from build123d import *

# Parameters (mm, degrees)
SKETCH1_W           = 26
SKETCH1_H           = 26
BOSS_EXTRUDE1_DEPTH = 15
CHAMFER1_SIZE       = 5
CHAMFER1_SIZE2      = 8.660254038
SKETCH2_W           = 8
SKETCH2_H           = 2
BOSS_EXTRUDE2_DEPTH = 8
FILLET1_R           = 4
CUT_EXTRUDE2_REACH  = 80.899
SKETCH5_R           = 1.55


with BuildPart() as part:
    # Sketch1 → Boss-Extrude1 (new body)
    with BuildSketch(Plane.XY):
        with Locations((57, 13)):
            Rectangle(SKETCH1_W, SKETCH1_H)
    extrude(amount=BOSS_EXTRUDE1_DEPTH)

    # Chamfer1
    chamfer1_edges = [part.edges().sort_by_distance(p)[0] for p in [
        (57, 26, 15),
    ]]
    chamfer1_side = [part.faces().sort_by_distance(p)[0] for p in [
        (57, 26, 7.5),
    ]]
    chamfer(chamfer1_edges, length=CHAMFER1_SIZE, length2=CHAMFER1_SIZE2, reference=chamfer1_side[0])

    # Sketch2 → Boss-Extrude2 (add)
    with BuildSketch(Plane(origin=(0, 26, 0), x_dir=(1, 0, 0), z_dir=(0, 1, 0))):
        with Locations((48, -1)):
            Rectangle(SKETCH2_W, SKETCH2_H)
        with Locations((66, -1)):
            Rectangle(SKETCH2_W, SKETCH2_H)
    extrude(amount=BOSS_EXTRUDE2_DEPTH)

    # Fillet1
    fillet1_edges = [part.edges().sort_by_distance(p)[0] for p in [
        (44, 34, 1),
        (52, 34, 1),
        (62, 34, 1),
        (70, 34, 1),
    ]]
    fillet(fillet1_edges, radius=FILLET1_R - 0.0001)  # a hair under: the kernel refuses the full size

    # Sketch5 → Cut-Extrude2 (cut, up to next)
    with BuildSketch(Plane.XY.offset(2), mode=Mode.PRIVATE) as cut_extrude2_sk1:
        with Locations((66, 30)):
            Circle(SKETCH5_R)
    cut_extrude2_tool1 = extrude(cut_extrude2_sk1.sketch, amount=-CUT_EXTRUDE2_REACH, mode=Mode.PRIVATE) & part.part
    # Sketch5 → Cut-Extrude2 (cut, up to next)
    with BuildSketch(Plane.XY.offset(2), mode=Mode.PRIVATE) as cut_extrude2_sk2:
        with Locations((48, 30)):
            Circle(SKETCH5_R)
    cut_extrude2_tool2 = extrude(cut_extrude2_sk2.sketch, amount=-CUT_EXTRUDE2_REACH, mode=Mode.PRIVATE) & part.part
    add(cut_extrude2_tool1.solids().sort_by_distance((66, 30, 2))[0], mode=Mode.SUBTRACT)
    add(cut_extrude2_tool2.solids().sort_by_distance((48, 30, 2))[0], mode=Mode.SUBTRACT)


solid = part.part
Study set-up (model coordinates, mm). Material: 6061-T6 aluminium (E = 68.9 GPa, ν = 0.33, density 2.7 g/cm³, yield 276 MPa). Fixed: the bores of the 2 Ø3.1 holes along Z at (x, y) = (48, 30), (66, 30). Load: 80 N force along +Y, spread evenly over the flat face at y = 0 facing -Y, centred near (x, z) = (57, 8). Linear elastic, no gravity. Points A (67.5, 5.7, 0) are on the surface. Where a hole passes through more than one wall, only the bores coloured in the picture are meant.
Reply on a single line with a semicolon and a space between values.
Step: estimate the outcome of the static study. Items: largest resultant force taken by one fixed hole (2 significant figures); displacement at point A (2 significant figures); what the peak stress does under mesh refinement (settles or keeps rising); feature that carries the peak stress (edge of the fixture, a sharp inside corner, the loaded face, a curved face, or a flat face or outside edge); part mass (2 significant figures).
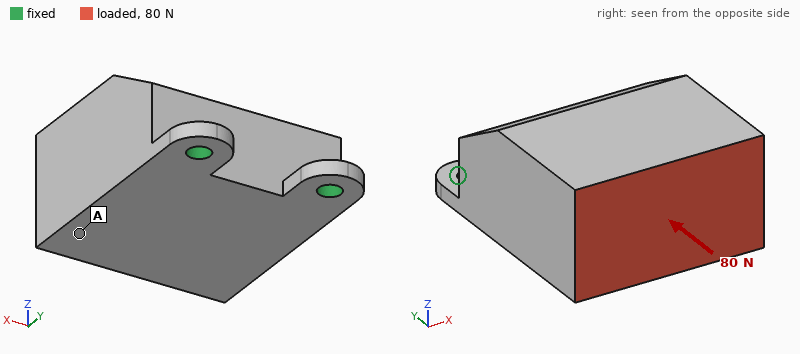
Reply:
40 N; 59 µm; keeps rising; edge of the fixture; 26 g
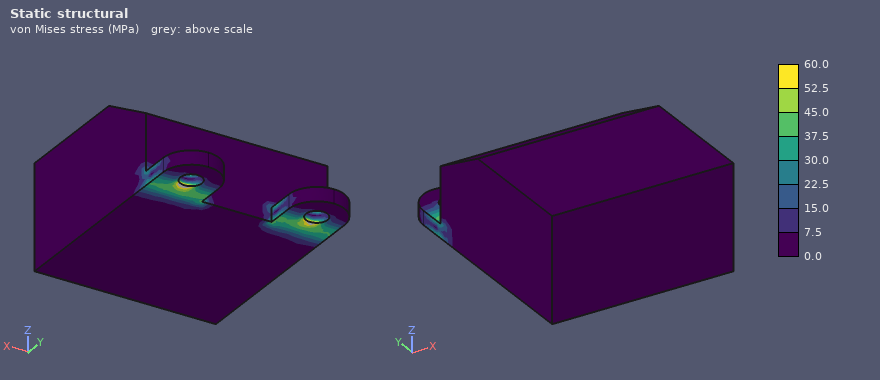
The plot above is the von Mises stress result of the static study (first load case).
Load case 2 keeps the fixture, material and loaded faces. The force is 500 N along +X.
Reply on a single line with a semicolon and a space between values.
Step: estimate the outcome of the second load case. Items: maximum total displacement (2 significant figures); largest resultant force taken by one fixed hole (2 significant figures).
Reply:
27 µm; 800 N
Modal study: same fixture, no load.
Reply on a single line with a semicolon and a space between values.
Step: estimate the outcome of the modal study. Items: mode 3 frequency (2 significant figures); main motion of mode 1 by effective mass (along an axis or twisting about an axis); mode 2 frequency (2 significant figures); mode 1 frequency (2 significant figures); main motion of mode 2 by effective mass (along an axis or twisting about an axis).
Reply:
8300 Hz; along Z; 6000 Hz; 750 Hz; along X
